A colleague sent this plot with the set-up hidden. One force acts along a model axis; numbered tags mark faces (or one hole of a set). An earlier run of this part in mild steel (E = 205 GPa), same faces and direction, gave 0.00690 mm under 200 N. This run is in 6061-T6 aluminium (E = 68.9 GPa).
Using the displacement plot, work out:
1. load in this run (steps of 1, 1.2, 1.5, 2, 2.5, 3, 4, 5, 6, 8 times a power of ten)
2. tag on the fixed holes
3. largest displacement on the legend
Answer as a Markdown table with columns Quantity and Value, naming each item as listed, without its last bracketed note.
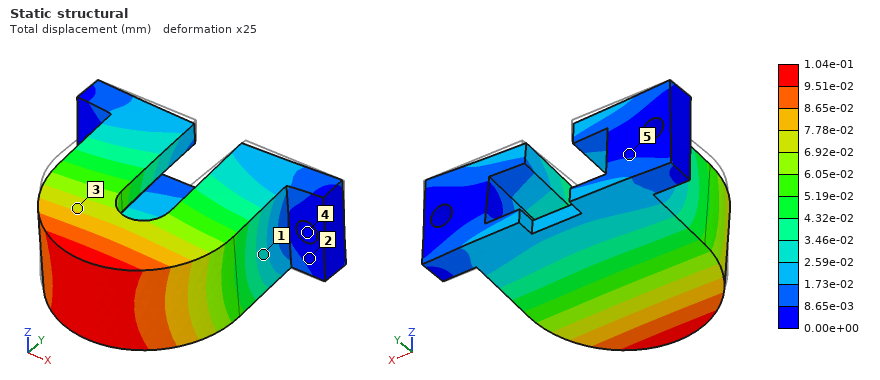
| Quantity | Value |
|---|---|
| load in this run | 1 kN |
| tag on the fixed holes | 4 |
| largest displacement on the legend | 1.04e-01 mm |
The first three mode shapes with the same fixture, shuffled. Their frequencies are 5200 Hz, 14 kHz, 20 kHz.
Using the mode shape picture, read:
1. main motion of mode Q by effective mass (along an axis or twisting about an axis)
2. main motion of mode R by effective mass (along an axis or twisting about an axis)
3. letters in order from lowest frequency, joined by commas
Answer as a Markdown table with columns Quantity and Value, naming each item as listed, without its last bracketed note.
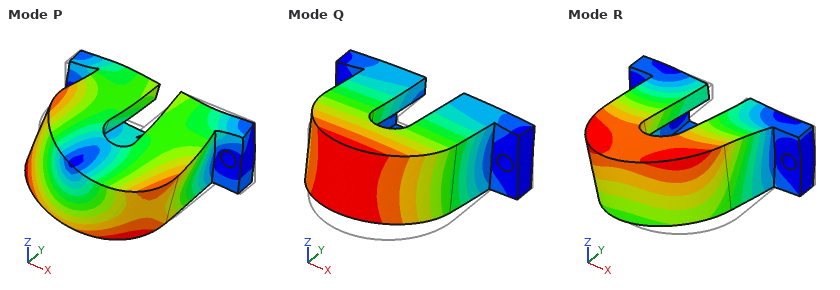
| Quantity | Value |
|---|---|
| main motion of mode Q by effective mass | along Z |
| main motion of mode R by effective mass | along X |
| letters in order from lowest frequency, joined by commas | Q, R, P |
